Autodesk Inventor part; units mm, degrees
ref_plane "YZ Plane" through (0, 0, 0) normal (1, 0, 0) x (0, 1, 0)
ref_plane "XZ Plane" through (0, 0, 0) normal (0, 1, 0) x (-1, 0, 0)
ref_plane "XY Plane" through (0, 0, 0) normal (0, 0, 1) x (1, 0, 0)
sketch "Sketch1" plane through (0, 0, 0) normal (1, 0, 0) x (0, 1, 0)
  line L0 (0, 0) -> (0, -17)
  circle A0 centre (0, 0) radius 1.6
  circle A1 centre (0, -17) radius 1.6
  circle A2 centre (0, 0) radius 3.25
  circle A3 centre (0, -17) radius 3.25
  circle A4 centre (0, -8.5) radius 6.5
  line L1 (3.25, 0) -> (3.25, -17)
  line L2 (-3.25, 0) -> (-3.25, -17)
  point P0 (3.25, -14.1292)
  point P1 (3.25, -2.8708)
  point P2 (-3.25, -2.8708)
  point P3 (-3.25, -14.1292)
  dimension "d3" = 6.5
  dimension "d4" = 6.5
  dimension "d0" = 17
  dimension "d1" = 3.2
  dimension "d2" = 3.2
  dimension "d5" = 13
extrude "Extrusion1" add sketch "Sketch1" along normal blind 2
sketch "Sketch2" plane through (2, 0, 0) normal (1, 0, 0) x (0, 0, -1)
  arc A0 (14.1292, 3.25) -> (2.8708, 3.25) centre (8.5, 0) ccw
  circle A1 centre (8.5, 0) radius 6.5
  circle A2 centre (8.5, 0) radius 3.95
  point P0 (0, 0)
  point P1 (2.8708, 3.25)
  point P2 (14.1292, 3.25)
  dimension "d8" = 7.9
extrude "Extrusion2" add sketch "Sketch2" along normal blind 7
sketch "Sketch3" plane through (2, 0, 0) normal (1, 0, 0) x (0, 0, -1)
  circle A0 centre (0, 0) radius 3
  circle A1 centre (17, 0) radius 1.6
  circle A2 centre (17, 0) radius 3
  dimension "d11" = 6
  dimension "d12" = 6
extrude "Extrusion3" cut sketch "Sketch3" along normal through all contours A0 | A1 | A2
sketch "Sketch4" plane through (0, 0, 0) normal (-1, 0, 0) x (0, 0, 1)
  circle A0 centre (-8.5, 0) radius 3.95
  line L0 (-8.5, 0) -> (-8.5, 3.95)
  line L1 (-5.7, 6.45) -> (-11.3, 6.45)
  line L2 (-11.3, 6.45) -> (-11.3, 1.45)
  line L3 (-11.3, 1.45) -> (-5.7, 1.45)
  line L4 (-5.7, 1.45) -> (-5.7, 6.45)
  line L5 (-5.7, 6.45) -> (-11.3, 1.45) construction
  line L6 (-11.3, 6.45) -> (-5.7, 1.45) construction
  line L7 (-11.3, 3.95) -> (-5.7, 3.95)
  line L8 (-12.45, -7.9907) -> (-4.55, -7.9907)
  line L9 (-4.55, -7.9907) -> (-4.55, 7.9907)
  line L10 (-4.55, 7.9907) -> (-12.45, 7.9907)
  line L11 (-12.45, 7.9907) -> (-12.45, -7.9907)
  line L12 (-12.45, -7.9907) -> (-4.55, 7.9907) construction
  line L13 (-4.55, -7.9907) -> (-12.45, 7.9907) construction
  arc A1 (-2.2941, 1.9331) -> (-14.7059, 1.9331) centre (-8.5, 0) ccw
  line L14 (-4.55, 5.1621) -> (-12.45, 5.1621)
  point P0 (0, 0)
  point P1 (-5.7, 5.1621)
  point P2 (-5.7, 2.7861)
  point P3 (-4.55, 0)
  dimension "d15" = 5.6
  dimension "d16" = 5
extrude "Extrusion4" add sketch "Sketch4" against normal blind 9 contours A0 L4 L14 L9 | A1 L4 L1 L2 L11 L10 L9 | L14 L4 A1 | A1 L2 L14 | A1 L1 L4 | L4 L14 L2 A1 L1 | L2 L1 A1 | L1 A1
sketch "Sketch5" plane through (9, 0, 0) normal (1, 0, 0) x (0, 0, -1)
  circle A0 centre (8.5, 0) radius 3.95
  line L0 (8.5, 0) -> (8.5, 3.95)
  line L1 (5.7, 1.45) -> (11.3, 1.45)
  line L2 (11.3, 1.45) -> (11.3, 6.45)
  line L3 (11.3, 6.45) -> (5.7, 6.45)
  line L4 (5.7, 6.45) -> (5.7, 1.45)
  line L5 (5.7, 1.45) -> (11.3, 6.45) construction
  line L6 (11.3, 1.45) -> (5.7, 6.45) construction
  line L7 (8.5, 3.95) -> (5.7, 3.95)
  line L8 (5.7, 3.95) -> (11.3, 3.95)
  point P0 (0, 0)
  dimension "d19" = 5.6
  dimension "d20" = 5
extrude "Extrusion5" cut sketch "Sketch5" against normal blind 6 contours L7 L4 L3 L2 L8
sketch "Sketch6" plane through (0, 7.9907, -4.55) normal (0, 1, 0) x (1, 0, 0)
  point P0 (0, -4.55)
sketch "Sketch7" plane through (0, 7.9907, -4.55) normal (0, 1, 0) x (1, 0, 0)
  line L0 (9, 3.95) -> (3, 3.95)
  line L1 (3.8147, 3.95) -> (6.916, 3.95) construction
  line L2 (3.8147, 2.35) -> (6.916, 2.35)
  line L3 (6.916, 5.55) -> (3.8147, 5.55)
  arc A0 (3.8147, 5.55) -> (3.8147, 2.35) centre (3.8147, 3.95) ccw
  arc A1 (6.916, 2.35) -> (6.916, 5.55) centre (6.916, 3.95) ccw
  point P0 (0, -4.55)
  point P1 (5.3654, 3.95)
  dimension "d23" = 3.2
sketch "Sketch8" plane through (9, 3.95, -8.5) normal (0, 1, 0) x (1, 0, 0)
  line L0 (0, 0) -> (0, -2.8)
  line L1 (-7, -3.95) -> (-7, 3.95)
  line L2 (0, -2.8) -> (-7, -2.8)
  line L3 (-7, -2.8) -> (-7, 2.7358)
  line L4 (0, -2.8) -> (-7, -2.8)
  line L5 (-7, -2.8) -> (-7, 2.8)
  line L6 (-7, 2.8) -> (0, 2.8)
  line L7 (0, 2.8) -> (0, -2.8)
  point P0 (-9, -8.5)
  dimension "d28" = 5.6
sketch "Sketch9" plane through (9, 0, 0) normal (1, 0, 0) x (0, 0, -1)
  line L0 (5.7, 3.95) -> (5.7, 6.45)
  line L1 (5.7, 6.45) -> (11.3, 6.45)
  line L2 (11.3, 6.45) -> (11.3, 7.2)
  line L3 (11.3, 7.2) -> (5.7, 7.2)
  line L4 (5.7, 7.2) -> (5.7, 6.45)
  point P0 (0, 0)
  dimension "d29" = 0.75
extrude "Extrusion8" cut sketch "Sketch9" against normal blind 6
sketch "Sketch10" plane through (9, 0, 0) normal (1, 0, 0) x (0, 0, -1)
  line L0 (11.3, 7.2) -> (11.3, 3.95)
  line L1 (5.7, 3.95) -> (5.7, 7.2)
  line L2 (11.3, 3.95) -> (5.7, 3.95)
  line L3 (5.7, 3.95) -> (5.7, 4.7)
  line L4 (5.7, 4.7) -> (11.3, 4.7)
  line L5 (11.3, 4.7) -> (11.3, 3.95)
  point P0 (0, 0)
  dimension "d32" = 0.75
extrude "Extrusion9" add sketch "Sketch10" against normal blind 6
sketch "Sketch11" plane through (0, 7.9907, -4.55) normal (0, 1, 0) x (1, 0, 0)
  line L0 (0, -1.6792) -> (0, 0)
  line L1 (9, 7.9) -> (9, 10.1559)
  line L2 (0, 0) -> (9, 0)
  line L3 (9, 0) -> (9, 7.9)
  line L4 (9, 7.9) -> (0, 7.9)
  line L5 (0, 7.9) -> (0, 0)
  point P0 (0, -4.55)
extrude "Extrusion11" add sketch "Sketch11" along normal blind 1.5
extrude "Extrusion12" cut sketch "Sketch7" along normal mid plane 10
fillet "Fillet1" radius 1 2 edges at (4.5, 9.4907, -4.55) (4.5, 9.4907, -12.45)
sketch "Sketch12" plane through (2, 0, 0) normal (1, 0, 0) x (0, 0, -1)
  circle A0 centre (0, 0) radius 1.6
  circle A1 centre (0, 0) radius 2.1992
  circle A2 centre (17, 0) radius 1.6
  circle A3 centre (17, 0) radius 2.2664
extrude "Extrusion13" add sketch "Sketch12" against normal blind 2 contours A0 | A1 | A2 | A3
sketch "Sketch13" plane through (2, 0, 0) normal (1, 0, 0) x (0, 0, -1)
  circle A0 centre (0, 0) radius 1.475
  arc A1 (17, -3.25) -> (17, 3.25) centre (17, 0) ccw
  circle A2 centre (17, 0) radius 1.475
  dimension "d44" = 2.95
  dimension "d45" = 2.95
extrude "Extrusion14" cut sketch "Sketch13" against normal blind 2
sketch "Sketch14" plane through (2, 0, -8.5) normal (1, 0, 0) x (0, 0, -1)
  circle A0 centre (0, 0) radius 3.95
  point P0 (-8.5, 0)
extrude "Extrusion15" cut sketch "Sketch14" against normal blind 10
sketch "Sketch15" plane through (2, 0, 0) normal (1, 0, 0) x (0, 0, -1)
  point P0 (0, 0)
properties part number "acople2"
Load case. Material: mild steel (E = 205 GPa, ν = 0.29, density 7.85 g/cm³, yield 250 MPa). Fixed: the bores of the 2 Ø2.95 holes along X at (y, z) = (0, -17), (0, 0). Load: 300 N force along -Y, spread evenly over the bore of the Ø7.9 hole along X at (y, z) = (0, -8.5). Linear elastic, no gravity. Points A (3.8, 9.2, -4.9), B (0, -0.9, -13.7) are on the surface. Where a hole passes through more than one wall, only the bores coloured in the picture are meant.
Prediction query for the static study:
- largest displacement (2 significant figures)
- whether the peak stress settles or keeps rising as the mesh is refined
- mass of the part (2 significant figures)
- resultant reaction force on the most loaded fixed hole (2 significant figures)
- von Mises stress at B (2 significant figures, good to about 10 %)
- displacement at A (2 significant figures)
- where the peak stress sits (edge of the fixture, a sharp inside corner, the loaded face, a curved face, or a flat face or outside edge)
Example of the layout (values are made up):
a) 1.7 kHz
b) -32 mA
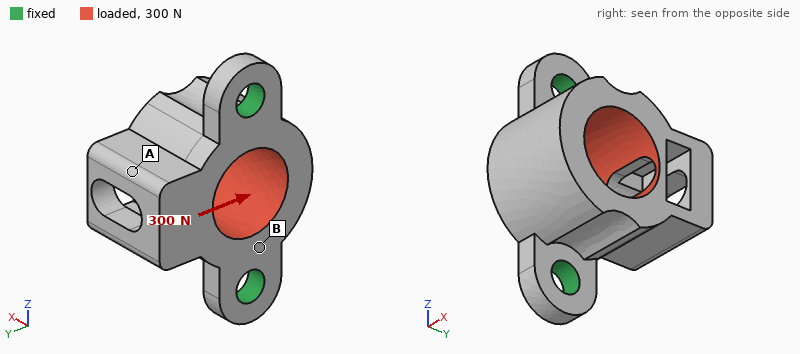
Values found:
a) 10.0 µm
b) keeps rising
c) 7.1 g
d) 150 N
e) 23 MPa
f) 7.6 µm
g) edge of the fixture
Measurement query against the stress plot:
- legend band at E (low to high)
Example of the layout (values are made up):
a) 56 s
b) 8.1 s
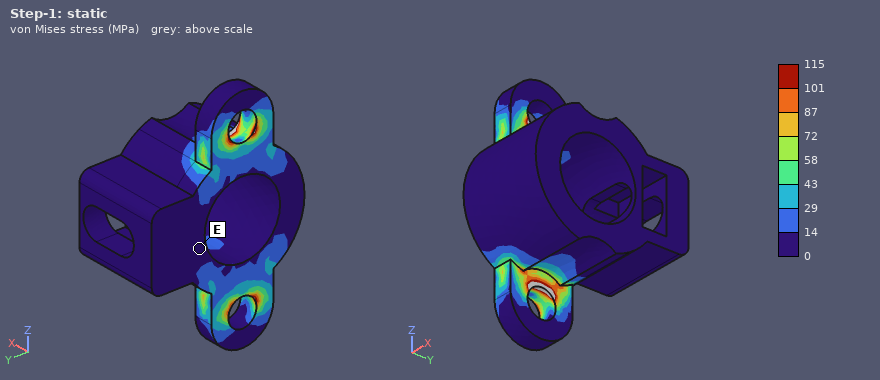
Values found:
a) 0 to 14 MPa
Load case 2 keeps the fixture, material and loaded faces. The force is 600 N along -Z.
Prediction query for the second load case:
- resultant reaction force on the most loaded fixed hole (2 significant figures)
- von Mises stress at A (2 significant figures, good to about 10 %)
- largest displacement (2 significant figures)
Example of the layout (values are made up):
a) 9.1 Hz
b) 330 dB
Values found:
a) 340 N
b) 7.0 MPa
c) 2.7 µm
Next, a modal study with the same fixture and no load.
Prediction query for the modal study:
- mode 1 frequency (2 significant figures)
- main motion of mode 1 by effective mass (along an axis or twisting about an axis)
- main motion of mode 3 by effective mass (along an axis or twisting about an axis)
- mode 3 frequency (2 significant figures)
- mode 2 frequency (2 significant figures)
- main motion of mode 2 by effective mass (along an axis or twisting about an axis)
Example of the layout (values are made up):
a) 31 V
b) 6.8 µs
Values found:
a) 11 kHz
b) along Y
c) along Z
d) 33 kHz
e) 31 kHz
f) along X
